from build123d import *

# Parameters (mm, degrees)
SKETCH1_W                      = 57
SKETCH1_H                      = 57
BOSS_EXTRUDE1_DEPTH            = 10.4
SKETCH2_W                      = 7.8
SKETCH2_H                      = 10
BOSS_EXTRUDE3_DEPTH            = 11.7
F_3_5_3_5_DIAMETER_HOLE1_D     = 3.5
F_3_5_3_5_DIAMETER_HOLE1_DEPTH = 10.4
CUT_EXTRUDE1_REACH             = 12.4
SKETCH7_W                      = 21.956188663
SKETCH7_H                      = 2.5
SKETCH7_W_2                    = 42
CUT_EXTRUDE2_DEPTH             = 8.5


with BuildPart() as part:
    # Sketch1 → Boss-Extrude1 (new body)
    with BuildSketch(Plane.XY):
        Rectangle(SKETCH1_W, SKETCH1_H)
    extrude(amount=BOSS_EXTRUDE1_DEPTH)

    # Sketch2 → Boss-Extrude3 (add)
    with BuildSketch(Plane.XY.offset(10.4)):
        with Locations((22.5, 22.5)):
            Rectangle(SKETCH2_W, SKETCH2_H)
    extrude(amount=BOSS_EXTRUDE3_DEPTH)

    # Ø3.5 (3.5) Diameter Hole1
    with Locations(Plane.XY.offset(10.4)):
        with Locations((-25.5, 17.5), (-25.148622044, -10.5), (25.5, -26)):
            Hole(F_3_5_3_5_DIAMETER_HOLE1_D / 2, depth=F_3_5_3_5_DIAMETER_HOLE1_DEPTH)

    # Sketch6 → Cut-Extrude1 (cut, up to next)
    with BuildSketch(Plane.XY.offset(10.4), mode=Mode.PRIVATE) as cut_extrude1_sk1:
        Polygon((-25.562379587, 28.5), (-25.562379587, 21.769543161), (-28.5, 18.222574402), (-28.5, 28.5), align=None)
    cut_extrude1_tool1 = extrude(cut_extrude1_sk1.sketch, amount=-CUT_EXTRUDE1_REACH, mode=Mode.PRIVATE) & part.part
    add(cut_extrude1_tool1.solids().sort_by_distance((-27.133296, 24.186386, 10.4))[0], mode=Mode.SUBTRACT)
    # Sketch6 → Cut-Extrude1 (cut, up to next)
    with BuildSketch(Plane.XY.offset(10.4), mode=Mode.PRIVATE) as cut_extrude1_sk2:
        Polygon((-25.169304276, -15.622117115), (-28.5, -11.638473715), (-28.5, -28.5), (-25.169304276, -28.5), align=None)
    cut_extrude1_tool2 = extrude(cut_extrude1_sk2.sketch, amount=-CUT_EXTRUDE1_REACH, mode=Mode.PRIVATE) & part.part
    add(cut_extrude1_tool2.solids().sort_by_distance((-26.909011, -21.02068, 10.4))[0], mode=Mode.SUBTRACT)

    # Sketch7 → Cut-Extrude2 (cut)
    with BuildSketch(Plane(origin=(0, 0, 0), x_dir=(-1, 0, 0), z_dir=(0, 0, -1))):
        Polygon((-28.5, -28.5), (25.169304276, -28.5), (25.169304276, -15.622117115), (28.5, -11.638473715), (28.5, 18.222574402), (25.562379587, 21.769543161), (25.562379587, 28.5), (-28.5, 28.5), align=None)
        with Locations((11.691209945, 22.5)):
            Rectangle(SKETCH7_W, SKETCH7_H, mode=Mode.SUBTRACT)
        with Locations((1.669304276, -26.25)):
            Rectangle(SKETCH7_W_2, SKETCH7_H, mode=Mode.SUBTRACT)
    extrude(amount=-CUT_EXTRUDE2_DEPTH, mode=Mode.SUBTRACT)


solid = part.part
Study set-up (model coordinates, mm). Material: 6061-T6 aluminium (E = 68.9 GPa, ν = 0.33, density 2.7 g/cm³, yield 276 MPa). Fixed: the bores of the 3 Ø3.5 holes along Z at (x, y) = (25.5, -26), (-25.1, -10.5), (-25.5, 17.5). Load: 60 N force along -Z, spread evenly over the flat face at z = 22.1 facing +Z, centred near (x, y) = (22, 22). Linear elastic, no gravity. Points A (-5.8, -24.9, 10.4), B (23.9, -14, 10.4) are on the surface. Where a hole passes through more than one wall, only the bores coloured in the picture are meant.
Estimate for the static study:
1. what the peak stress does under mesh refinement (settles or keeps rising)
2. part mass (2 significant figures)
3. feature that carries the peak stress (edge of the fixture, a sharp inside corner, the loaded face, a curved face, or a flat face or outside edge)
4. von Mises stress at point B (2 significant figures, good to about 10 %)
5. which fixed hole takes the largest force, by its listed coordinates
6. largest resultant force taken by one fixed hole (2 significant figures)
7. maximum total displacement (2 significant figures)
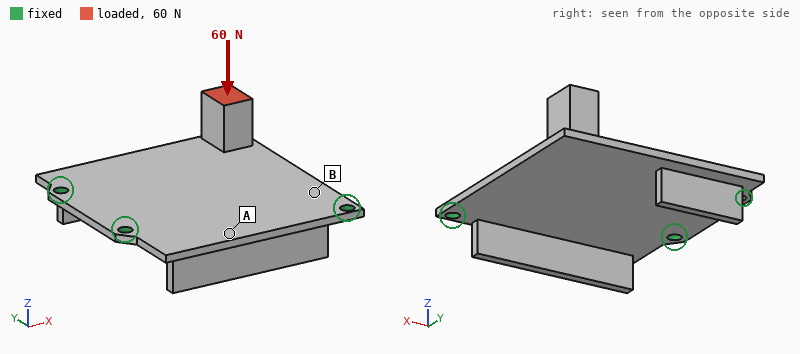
keeps rising
22 g
edge of the fixture
44 MPa
(-25.5, 17.5)
58 N
0.76 mm
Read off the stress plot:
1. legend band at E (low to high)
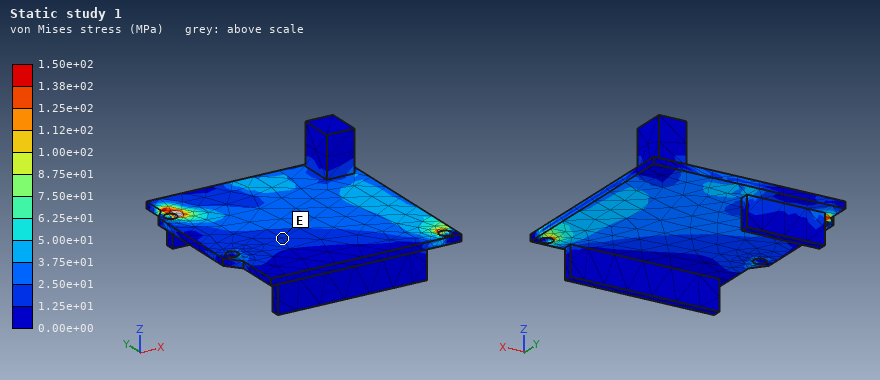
1.25e+01 to 2.50e+01 MPa
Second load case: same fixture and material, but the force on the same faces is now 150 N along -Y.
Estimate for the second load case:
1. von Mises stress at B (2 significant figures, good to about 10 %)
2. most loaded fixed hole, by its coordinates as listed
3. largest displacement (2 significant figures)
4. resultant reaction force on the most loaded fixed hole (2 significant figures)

21 MPa
(25.5, -26)
0.71 mm
110 N
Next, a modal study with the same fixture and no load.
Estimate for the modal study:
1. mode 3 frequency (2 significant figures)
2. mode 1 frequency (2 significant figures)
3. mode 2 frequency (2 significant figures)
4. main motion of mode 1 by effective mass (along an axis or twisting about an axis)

2700 Hz
730 Hz
2700 Hz
along Z
